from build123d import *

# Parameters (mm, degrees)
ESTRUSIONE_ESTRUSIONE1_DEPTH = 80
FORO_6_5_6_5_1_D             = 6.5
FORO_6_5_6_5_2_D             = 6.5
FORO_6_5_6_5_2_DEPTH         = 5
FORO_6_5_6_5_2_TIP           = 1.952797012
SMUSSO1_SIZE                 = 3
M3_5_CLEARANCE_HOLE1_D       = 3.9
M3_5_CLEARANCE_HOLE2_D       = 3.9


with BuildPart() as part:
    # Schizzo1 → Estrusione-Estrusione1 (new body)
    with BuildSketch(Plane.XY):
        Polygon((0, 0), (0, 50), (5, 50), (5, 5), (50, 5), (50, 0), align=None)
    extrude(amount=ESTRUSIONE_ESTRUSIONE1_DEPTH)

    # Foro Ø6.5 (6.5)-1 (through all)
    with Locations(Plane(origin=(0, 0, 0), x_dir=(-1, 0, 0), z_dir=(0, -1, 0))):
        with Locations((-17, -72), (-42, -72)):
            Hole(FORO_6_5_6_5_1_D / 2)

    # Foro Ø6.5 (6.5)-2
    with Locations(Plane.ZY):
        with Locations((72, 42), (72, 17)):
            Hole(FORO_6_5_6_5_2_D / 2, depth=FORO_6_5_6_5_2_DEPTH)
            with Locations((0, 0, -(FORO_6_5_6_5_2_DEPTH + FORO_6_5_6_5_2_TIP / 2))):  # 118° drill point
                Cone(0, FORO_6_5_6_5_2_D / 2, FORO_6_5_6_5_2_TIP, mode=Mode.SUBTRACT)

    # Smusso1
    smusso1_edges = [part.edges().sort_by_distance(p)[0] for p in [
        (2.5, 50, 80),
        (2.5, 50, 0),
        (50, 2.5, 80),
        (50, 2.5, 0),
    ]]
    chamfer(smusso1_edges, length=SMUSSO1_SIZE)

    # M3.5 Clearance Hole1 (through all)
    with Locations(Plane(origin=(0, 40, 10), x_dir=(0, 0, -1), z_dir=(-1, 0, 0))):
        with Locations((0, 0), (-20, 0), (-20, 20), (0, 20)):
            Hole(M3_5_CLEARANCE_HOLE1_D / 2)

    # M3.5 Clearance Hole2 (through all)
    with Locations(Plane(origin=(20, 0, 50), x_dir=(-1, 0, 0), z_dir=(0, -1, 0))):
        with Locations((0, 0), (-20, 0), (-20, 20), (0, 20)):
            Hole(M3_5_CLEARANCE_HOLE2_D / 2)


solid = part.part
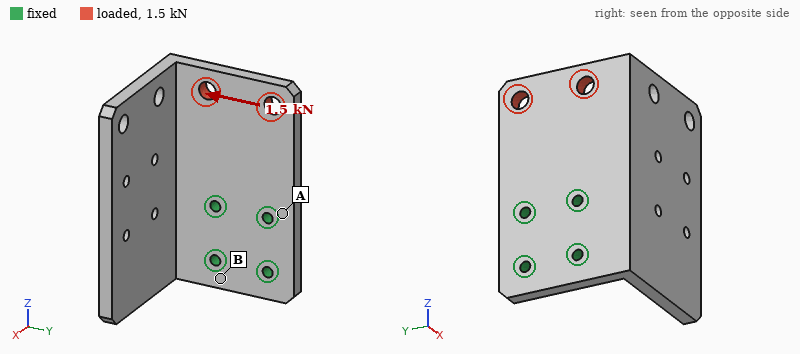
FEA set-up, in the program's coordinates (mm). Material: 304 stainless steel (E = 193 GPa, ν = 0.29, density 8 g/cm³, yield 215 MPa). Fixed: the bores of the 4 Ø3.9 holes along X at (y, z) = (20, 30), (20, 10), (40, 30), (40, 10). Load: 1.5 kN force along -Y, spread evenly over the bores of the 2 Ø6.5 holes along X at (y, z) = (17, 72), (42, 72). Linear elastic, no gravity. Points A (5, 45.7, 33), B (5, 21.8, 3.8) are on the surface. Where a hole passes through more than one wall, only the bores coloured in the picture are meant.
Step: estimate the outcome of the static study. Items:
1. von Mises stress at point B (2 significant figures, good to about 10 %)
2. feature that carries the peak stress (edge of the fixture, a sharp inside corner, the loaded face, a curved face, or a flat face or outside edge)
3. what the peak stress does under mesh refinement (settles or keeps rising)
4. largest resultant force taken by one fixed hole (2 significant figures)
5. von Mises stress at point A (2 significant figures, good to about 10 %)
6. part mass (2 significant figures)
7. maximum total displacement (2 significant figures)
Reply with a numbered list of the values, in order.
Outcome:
1. 7.3 MPa
2. edge of the fixture
3. keeps rising
4. 1.9 kN
5. 21 MPa
6. 290 g
7. 13 µm
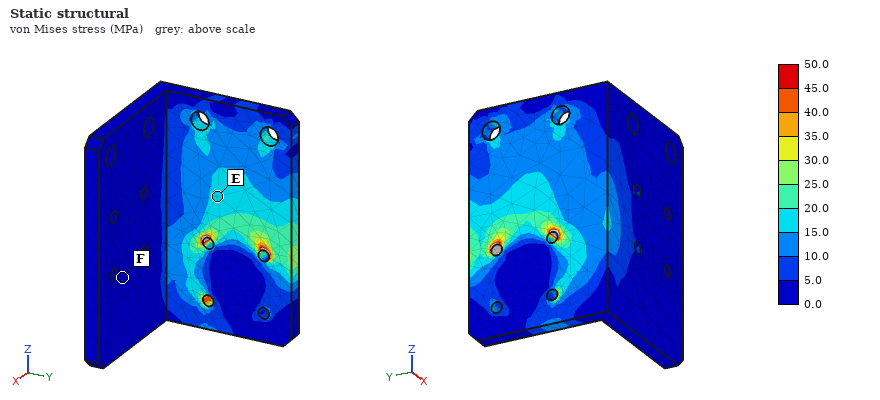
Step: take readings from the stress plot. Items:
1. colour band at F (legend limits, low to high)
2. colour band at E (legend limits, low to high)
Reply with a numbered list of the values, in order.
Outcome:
1. 0.0 to 5.0 MPa
2. 15.0 to 20.0 MPa
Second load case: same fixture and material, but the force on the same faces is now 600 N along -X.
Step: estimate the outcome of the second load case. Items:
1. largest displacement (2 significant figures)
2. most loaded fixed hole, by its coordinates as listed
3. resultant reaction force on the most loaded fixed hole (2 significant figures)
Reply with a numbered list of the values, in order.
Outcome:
1. 0.12 mm
2. (20, 30)
3. 950 N
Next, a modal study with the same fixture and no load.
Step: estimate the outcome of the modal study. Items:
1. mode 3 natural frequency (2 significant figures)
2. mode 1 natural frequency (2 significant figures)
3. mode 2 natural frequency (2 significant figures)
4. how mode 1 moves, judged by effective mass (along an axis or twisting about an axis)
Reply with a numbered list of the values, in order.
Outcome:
1. 2400 Hz
2. 1000 Hz
3. 1400 Hz
4. along Y
